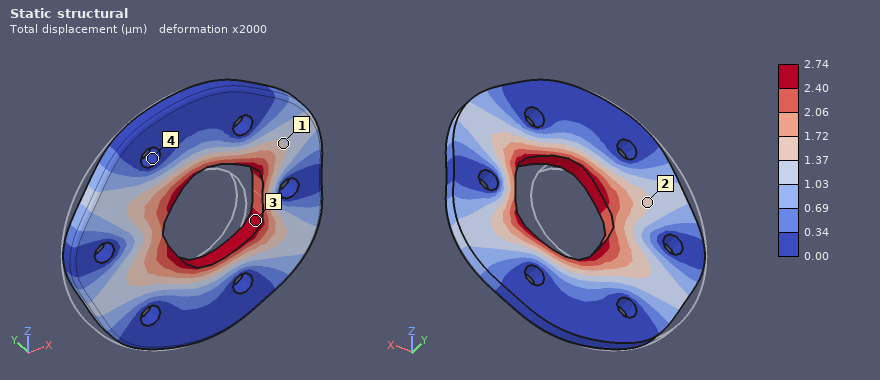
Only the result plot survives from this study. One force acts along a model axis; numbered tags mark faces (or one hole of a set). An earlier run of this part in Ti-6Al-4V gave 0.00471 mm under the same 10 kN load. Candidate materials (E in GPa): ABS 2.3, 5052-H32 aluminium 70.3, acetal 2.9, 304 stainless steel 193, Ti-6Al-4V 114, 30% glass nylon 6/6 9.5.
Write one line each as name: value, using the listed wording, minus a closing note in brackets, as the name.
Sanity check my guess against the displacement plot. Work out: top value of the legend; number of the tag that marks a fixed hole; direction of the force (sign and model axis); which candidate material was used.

top value of the legend: 2.74 µm
number of the tag that marks a fixed hole: 4
direction of the force: +X
which candidate material was used: 304 stainless steel
